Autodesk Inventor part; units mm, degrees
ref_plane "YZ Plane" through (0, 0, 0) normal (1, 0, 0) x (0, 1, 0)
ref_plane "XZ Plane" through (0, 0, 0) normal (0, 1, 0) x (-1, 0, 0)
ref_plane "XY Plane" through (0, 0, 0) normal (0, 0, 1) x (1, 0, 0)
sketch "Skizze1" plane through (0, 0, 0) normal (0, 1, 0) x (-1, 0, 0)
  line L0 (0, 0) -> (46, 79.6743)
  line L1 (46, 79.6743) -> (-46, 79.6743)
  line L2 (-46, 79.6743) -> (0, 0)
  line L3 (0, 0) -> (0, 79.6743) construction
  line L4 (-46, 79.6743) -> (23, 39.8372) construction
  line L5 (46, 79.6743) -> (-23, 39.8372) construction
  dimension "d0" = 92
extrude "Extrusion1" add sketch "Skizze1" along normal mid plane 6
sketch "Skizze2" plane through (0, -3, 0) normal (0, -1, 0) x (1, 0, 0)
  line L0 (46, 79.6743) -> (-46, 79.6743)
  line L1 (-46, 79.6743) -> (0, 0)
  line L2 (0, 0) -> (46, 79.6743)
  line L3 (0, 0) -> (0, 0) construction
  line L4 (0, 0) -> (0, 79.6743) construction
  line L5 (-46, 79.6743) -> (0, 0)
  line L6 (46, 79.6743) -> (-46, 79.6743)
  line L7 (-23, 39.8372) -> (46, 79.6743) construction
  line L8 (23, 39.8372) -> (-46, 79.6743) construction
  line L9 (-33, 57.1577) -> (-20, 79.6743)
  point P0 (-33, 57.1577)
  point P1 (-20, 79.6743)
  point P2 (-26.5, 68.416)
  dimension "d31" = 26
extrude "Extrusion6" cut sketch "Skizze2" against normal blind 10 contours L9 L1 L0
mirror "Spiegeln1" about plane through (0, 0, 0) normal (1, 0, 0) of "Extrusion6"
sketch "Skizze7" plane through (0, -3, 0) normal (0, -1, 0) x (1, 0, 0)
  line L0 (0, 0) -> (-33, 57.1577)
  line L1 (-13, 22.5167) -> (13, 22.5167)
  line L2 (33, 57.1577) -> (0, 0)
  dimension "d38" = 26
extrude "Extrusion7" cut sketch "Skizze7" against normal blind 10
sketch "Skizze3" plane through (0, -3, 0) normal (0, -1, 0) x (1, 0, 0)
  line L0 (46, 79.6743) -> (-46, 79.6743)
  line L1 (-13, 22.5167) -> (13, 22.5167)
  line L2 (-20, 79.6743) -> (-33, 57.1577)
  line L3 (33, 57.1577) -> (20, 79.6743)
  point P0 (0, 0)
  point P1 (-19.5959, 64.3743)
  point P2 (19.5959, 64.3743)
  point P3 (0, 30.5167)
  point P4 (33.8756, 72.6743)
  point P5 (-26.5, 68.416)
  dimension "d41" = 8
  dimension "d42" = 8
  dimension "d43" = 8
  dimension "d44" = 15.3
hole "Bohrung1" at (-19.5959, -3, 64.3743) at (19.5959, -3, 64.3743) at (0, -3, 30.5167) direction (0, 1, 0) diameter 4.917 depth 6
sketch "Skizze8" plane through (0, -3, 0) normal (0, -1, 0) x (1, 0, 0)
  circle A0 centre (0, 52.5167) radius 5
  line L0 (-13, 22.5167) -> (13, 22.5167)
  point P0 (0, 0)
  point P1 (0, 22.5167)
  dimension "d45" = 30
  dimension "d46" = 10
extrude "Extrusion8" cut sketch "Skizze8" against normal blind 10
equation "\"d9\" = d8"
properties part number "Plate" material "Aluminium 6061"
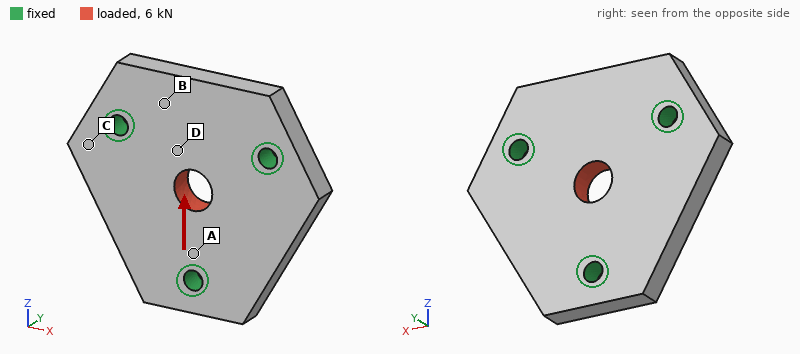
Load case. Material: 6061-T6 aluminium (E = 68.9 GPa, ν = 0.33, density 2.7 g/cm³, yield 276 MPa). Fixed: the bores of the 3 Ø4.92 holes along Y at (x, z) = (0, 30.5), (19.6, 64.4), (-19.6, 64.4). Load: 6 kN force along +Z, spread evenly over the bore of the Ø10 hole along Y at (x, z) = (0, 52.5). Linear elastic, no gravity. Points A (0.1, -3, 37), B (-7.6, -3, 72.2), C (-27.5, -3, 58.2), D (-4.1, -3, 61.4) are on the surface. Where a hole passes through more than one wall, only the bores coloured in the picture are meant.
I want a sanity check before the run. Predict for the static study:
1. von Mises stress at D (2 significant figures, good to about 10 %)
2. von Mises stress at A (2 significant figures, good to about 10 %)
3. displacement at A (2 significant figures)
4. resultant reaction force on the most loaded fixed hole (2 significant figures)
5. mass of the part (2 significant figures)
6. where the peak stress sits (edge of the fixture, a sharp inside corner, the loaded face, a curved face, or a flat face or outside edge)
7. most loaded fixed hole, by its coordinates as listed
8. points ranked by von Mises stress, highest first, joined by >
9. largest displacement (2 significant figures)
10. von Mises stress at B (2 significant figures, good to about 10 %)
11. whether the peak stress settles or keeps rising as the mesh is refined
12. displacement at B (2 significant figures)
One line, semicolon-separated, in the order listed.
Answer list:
22 MPa; 37 MPa; 2.3 µm; 2.3 kN; 43 g; edge of the fixture; (0, 30.5); A > D > B > C; 11 µm; 13 MPa; keeps rising; 5.6 µm
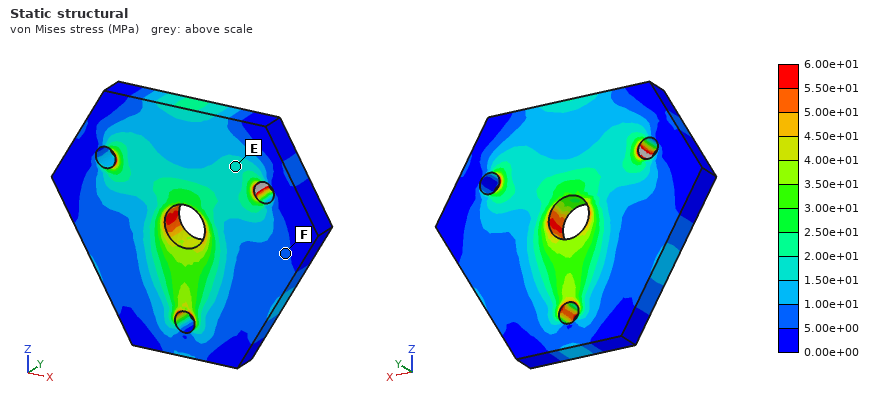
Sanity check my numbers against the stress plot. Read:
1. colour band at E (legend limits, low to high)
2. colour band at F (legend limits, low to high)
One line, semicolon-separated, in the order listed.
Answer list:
1.50e+01 to 2.00e+01 MPa; 5.00e+00 to 1.00e+01 MPa
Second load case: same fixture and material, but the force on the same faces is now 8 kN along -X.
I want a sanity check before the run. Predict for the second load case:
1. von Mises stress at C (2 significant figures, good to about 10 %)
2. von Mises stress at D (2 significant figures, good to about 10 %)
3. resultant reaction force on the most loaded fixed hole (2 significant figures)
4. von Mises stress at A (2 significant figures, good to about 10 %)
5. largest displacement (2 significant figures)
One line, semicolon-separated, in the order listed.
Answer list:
7.4 MPa; 31 MPa; 2.8 kN; 15 MPa; 14 µm
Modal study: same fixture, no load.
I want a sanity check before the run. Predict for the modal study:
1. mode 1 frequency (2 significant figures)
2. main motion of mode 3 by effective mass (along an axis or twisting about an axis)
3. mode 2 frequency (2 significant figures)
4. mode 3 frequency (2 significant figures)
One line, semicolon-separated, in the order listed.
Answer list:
13 kHz; along Y; 13 kHz; 15 kHz
